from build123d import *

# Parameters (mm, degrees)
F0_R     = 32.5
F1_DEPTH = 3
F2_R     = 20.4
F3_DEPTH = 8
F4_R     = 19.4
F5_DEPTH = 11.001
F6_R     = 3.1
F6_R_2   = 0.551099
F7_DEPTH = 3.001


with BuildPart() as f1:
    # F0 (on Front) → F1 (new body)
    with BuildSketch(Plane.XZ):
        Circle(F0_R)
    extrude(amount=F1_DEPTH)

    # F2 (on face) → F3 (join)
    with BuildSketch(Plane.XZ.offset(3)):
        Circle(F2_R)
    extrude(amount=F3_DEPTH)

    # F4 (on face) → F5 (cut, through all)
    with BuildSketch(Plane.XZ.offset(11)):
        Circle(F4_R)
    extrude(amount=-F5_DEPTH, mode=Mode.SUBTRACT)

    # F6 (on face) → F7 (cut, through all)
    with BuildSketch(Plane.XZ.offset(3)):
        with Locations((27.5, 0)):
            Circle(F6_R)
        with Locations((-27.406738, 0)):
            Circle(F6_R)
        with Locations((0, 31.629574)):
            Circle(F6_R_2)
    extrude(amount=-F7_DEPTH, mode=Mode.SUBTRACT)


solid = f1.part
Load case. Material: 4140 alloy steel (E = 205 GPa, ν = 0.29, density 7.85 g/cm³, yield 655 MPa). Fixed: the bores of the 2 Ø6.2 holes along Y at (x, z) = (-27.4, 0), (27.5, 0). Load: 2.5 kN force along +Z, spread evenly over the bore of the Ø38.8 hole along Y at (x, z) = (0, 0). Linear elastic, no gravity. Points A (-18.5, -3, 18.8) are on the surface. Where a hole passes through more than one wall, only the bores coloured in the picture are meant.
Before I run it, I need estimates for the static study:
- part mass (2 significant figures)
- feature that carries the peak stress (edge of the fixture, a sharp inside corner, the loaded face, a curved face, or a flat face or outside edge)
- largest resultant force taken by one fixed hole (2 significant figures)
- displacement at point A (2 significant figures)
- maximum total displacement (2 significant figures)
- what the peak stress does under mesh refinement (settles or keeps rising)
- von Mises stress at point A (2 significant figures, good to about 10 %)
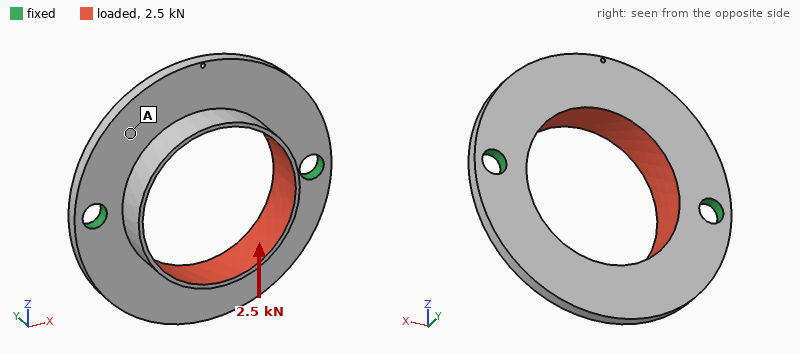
57 g
edge of the fixture
1.3 kN
37 µm
87 µm
keeps rising
25 MPa
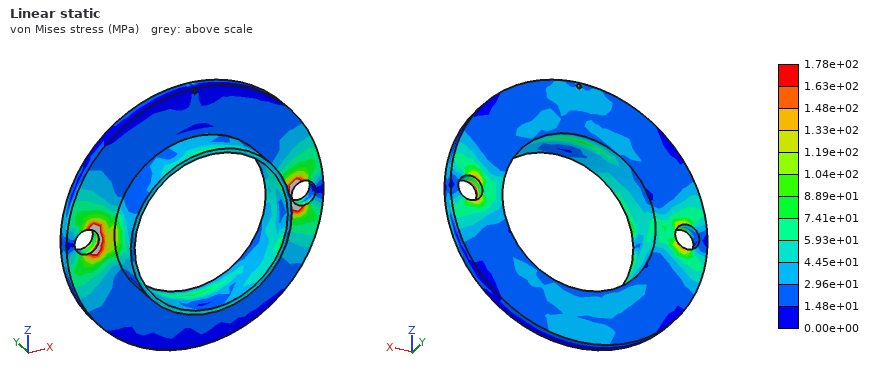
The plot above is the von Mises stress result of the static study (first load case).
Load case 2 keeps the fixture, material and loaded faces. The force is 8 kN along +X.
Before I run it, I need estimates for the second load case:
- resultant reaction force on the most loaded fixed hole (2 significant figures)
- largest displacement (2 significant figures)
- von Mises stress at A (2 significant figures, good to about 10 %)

4.1 kN
43 µm
46 MPa
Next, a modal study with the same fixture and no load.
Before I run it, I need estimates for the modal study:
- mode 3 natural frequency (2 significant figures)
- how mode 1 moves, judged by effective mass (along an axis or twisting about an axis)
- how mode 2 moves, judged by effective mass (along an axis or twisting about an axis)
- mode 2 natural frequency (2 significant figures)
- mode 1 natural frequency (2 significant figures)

6200 Hz
twisting about X
along Y
2700 Hz
2300 Hz
